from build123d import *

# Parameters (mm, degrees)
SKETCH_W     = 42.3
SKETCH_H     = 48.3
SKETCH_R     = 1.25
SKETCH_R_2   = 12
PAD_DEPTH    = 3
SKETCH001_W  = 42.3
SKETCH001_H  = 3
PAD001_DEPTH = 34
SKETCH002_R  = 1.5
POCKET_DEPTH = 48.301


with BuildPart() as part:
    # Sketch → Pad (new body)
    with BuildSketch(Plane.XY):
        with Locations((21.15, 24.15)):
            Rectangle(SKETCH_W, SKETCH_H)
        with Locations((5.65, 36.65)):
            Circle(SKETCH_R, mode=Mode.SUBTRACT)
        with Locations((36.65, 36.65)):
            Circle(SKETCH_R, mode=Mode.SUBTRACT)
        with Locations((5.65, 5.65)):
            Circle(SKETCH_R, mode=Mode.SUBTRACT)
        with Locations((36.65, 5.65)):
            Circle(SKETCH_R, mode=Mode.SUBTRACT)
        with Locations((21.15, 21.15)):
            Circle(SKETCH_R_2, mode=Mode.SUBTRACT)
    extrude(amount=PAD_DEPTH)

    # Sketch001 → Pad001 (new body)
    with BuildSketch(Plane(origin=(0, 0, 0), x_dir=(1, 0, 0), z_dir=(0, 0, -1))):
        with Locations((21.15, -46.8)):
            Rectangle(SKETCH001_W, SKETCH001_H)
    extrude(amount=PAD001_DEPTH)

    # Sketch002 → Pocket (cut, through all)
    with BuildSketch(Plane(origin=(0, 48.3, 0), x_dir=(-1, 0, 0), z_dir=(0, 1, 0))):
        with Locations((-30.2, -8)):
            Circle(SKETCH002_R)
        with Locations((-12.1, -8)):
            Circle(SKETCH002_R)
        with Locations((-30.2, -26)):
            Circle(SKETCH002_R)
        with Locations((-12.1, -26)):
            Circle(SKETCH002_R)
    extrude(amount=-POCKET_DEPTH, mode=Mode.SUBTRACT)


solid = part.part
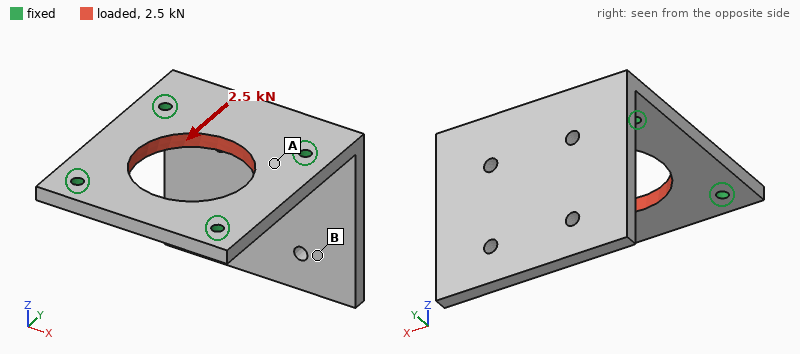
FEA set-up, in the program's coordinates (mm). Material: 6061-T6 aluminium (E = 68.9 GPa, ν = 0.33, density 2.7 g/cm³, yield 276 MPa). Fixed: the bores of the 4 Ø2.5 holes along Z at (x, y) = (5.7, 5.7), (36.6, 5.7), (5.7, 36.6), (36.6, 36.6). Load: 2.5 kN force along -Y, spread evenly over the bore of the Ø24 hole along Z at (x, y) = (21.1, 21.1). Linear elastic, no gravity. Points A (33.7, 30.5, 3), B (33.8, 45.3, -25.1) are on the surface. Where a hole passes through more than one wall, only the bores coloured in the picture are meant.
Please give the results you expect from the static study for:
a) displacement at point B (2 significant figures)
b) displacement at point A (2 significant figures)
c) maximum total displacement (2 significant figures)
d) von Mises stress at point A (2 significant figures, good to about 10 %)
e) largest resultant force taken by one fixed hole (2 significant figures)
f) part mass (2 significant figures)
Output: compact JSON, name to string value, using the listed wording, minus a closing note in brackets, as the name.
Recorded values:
{"displacement at point B": "3.1 µm", "displacement at point A": "2.0 µm", "maximum total displacement": "9.5 µm", "von Mises stress at point A": "17 MPa", "largest resultant force taken by one fixed hole": "630 N", "part mass": "24 g"}
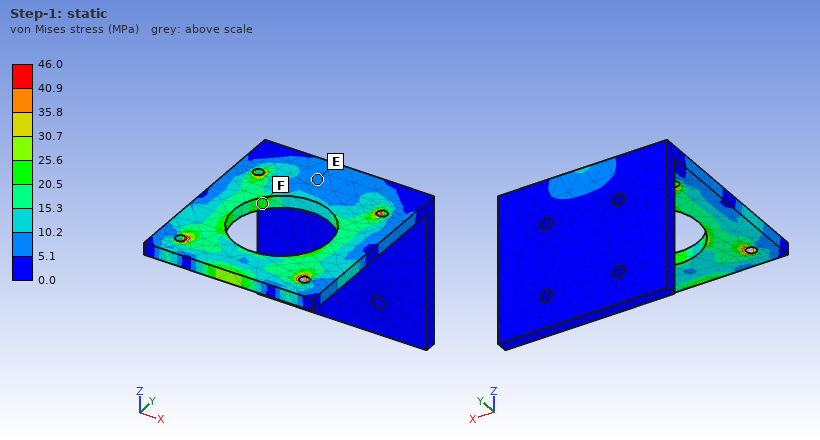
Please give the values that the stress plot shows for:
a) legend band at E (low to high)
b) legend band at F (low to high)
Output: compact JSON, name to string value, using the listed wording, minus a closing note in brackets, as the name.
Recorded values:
{"legend band at E": "5.1 to 10.2 MPa", "legend band at F": "20.5 to 25.6 MPa"}
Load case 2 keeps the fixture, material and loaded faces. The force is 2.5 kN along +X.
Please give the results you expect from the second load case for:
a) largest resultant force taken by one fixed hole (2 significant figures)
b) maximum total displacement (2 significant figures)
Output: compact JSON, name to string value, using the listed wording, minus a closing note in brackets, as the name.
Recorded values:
{"largest resultant force taken by one fixed hole": "650 N", "maximum total displacement": "8.5 µm"}
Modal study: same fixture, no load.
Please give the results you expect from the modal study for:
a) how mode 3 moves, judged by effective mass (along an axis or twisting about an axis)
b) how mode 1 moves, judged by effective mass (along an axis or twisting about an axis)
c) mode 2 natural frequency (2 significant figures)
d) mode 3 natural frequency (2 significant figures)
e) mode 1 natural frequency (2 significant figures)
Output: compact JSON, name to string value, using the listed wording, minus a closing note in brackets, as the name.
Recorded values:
{"how mode 3 moves, judged by effective mass": "along X", "how mode 1 moves, judged by effective mass": "along Y", "mode 2 natural frequency": "3300 Hz", "mode 3 natural frequency": "4900 Hz", "mode 1 natural frequency": "1300 Hz"}
